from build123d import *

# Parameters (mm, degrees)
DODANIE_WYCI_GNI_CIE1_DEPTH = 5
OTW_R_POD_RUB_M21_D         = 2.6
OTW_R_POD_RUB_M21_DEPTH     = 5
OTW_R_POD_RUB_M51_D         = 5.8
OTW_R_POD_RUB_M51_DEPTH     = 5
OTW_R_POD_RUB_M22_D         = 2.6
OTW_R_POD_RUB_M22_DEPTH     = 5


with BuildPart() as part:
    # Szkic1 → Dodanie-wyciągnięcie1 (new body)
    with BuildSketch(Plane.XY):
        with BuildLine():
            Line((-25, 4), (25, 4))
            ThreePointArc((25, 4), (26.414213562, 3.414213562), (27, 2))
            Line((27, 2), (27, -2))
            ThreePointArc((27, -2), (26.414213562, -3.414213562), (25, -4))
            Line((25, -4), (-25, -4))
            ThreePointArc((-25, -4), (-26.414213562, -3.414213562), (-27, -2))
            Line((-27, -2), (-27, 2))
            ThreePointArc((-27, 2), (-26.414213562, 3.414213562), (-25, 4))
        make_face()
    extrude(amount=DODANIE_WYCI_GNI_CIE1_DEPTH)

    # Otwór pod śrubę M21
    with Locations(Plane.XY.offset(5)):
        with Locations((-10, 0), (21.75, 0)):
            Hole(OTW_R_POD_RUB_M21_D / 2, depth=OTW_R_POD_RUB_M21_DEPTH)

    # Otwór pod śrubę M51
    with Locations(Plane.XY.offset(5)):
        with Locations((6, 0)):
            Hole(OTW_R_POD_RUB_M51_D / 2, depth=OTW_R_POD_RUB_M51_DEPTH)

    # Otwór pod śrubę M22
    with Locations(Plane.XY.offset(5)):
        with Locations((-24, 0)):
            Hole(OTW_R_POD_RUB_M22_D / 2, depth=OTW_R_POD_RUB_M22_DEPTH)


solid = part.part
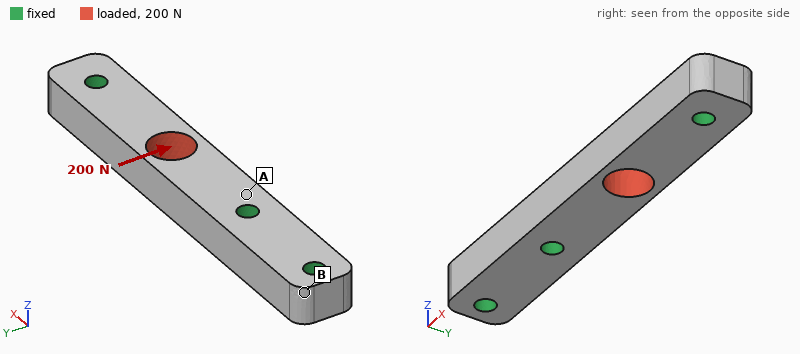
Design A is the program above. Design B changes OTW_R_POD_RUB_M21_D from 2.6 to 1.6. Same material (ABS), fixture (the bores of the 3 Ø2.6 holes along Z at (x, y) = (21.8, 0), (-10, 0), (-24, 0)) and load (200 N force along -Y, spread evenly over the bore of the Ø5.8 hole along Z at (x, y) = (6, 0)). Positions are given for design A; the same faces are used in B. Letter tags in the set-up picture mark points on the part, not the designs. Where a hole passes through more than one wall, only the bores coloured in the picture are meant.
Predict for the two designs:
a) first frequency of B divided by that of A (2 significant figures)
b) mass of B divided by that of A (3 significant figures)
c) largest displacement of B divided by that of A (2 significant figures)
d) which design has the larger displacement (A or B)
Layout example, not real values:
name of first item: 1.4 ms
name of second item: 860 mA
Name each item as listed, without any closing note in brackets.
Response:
first frequency of B divided by that of A: 0.91
mass of B divided by that of A: 1.02
largest displacement of B divided by that of A: 1.3
which design has the larger displacement: B
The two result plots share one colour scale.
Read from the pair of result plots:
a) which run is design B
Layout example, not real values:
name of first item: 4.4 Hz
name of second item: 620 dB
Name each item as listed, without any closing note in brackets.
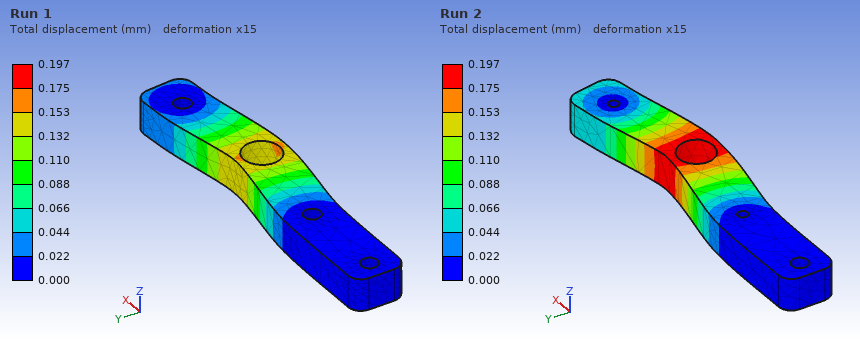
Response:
which run is design B: Run 2
